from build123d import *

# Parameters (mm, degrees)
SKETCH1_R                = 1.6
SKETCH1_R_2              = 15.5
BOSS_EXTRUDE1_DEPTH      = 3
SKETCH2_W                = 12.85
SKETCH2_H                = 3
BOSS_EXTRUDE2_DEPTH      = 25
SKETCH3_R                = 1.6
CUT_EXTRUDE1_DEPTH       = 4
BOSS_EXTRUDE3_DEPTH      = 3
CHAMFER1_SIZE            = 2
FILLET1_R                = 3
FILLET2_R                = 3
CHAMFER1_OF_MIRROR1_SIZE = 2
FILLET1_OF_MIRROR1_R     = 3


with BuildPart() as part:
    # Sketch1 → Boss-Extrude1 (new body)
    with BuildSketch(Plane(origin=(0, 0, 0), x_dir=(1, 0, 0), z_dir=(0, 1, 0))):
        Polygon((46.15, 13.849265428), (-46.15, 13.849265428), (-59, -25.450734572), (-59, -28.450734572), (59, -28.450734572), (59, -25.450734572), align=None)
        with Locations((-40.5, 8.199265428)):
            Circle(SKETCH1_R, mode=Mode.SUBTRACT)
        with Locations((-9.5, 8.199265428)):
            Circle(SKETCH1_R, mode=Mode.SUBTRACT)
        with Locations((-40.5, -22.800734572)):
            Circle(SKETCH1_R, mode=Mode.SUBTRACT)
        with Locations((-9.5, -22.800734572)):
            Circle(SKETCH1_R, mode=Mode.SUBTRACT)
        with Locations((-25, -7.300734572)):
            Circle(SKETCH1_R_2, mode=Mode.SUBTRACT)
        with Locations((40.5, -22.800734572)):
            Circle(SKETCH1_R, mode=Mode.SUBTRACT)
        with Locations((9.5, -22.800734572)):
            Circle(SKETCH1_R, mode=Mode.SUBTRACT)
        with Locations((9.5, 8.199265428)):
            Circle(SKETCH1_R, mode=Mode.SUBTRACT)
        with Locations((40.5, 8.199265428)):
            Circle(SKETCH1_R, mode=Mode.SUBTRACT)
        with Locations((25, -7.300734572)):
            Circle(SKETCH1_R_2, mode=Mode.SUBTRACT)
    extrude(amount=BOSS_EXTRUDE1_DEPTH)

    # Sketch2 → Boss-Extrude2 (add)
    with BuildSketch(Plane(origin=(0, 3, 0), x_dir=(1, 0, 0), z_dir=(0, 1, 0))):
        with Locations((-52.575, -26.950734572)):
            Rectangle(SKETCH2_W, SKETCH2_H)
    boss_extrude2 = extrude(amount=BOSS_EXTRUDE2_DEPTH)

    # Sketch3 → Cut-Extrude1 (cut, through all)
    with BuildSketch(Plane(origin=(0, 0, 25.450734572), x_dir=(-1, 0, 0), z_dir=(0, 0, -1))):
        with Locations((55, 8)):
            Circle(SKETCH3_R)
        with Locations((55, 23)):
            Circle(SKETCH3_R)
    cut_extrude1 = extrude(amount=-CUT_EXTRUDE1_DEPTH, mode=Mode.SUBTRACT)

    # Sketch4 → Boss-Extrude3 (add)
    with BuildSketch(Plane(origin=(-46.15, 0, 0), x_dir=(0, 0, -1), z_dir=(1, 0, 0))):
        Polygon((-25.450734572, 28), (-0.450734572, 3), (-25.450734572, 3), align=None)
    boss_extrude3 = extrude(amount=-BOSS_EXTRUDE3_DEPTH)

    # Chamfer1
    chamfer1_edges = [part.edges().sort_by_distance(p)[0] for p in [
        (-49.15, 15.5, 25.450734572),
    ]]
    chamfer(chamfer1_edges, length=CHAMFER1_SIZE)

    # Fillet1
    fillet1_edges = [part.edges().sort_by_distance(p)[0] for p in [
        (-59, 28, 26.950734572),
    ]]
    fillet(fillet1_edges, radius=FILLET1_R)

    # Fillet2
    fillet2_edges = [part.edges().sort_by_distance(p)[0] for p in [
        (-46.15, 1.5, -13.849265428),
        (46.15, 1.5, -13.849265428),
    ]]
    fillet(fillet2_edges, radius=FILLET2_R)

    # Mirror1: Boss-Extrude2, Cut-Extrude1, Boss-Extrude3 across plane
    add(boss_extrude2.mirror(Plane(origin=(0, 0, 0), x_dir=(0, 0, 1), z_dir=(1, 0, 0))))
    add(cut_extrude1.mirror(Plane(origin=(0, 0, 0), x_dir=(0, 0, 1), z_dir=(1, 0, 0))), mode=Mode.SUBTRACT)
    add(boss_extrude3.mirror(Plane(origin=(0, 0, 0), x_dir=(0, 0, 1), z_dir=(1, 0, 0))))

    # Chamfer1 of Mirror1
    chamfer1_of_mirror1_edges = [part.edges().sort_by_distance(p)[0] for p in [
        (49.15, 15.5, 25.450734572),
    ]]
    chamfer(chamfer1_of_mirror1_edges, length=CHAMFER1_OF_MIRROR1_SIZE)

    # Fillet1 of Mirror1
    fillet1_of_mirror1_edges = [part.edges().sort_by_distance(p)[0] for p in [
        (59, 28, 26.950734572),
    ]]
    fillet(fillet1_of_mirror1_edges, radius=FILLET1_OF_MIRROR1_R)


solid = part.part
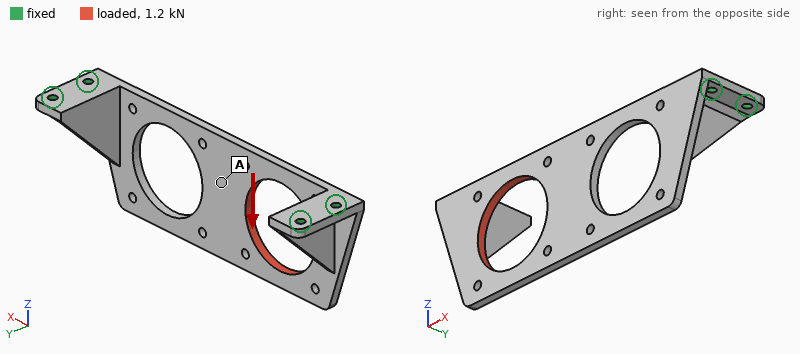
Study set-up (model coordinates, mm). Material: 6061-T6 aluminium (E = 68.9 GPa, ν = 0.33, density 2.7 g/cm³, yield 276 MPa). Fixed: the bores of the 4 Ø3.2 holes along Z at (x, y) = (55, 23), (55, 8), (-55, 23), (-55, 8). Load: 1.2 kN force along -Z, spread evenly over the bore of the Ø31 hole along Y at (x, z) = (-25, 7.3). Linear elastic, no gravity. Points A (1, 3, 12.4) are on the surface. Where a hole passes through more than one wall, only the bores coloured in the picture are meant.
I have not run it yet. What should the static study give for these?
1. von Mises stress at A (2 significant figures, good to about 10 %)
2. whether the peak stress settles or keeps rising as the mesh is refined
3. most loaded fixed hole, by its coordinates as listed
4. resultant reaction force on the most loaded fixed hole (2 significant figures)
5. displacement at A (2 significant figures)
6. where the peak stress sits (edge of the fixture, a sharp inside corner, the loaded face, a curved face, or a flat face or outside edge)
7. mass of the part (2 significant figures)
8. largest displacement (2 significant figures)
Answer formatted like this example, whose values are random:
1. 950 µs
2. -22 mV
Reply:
1. 8.1 MPa
2. keeps rising
3. (-55, 8)
4. 1.2 kN
5. 0.080 mm
6. edge of the fixture
7. 34 g
8. 0.10 mm
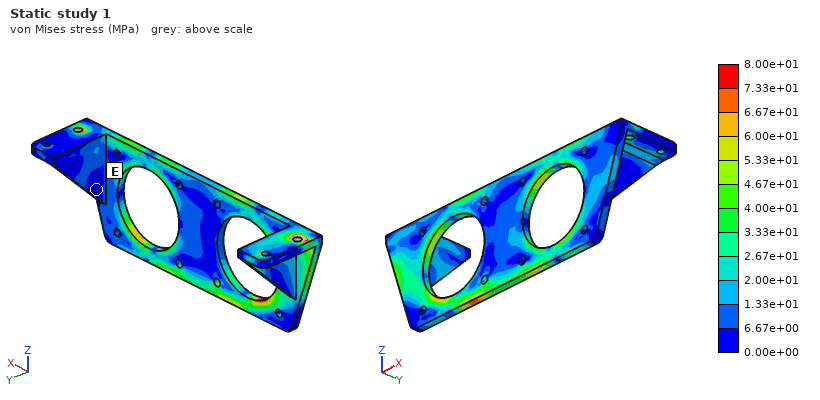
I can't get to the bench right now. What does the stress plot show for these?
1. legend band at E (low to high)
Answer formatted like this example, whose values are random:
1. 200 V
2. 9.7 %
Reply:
1. 0.00e+00 to 6.67e+00 MPa
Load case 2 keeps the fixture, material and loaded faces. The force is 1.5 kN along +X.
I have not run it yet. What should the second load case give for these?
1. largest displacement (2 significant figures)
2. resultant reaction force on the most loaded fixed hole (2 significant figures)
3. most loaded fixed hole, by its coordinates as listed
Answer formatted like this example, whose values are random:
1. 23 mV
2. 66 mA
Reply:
1. 58 µm
2. 1.2 kN
3. (-55, 8)
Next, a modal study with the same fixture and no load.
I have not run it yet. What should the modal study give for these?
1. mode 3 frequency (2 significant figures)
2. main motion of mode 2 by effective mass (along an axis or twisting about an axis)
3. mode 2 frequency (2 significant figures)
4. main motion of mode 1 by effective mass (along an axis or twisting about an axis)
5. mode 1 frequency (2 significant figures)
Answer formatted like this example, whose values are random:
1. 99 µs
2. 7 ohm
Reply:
1. 3400 Hz
2. twisting about X
3. 2000 Hz
4. along Y
5. 1200 Hz
